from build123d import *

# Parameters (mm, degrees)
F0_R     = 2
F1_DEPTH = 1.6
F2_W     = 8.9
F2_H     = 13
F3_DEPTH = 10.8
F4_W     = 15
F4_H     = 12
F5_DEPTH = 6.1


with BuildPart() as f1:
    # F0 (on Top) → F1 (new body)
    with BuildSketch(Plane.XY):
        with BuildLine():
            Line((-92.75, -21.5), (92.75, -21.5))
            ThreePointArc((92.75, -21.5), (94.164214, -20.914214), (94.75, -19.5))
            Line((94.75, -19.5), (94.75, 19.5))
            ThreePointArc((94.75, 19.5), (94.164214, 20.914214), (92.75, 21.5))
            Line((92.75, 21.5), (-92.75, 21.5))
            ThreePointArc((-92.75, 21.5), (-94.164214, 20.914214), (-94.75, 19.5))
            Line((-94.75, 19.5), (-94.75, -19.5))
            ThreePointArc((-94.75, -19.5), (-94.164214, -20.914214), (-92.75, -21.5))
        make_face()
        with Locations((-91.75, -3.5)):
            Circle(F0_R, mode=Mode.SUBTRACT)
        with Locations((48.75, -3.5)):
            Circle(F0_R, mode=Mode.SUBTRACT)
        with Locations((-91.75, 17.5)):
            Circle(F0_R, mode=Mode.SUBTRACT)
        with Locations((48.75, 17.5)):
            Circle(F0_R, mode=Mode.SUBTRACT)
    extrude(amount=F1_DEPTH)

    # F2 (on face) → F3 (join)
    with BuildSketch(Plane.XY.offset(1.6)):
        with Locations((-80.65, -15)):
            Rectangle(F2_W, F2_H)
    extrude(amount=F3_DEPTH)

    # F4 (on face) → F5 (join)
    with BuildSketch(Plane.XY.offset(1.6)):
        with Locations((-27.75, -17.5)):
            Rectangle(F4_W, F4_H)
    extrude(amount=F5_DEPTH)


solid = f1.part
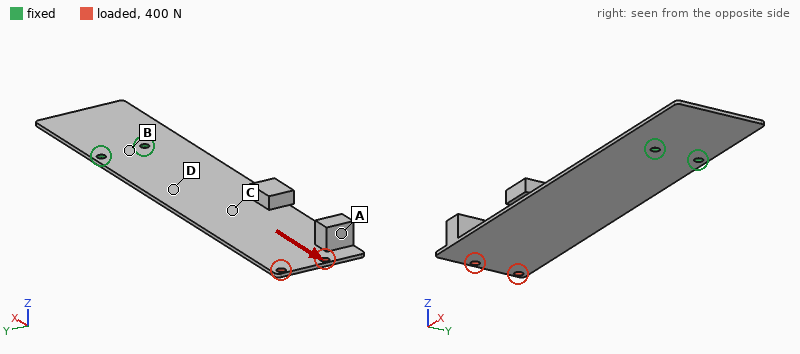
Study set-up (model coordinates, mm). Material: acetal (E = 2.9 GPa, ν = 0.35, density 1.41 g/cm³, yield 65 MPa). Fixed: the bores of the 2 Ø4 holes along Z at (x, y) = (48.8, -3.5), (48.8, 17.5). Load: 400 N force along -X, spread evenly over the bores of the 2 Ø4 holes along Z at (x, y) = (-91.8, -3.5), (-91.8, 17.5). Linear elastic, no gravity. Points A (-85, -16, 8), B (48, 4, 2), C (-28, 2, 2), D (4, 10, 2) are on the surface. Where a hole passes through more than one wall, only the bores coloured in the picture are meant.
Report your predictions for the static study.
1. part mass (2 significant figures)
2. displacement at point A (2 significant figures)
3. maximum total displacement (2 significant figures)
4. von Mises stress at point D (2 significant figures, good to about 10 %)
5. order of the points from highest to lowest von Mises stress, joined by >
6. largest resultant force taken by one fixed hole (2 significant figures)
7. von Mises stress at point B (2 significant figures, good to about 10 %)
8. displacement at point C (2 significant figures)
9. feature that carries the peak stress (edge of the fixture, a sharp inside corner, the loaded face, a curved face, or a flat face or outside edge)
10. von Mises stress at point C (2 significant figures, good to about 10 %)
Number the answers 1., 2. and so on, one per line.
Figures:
1. 22 g
2. 0.75 mm
3. 1.1 mm
4. 8.6 MPa
5. D > C > B > A
6. 200 N
7. 3.3 MPa
8. 0.29 mm
9. the loaded face
10. 6.1 MPa
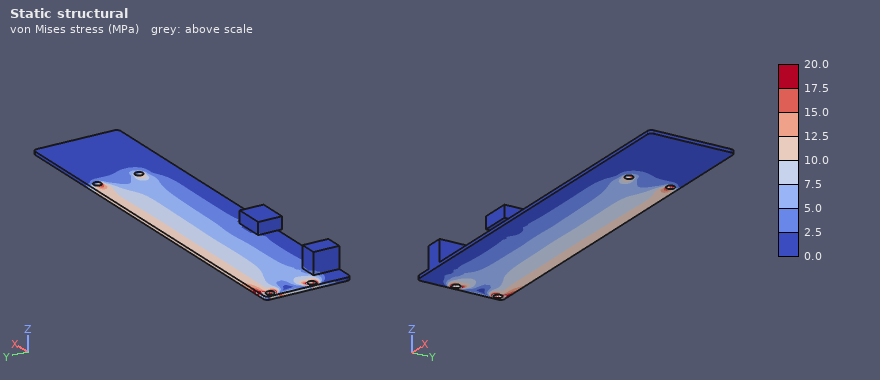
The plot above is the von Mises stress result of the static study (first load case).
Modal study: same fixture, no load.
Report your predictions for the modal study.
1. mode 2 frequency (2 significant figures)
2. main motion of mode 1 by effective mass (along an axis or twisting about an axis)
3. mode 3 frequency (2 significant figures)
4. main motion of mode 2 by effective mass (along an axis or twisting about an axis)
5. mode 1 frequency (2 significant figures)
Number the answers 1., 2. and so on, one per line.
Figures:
1. 99 Hz
2. along Z
3. 100 Hz
4. twisting about X
5. 15 Hz
